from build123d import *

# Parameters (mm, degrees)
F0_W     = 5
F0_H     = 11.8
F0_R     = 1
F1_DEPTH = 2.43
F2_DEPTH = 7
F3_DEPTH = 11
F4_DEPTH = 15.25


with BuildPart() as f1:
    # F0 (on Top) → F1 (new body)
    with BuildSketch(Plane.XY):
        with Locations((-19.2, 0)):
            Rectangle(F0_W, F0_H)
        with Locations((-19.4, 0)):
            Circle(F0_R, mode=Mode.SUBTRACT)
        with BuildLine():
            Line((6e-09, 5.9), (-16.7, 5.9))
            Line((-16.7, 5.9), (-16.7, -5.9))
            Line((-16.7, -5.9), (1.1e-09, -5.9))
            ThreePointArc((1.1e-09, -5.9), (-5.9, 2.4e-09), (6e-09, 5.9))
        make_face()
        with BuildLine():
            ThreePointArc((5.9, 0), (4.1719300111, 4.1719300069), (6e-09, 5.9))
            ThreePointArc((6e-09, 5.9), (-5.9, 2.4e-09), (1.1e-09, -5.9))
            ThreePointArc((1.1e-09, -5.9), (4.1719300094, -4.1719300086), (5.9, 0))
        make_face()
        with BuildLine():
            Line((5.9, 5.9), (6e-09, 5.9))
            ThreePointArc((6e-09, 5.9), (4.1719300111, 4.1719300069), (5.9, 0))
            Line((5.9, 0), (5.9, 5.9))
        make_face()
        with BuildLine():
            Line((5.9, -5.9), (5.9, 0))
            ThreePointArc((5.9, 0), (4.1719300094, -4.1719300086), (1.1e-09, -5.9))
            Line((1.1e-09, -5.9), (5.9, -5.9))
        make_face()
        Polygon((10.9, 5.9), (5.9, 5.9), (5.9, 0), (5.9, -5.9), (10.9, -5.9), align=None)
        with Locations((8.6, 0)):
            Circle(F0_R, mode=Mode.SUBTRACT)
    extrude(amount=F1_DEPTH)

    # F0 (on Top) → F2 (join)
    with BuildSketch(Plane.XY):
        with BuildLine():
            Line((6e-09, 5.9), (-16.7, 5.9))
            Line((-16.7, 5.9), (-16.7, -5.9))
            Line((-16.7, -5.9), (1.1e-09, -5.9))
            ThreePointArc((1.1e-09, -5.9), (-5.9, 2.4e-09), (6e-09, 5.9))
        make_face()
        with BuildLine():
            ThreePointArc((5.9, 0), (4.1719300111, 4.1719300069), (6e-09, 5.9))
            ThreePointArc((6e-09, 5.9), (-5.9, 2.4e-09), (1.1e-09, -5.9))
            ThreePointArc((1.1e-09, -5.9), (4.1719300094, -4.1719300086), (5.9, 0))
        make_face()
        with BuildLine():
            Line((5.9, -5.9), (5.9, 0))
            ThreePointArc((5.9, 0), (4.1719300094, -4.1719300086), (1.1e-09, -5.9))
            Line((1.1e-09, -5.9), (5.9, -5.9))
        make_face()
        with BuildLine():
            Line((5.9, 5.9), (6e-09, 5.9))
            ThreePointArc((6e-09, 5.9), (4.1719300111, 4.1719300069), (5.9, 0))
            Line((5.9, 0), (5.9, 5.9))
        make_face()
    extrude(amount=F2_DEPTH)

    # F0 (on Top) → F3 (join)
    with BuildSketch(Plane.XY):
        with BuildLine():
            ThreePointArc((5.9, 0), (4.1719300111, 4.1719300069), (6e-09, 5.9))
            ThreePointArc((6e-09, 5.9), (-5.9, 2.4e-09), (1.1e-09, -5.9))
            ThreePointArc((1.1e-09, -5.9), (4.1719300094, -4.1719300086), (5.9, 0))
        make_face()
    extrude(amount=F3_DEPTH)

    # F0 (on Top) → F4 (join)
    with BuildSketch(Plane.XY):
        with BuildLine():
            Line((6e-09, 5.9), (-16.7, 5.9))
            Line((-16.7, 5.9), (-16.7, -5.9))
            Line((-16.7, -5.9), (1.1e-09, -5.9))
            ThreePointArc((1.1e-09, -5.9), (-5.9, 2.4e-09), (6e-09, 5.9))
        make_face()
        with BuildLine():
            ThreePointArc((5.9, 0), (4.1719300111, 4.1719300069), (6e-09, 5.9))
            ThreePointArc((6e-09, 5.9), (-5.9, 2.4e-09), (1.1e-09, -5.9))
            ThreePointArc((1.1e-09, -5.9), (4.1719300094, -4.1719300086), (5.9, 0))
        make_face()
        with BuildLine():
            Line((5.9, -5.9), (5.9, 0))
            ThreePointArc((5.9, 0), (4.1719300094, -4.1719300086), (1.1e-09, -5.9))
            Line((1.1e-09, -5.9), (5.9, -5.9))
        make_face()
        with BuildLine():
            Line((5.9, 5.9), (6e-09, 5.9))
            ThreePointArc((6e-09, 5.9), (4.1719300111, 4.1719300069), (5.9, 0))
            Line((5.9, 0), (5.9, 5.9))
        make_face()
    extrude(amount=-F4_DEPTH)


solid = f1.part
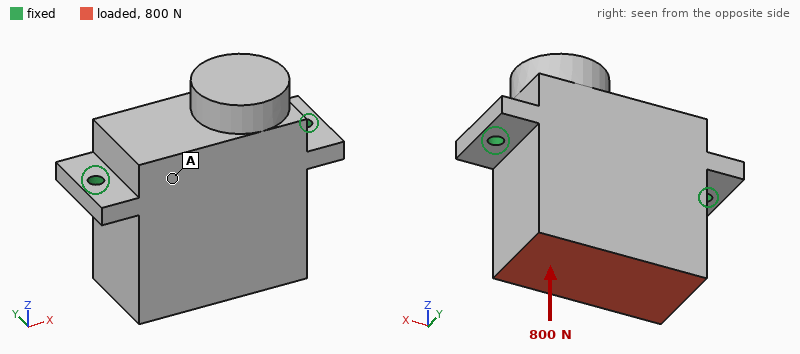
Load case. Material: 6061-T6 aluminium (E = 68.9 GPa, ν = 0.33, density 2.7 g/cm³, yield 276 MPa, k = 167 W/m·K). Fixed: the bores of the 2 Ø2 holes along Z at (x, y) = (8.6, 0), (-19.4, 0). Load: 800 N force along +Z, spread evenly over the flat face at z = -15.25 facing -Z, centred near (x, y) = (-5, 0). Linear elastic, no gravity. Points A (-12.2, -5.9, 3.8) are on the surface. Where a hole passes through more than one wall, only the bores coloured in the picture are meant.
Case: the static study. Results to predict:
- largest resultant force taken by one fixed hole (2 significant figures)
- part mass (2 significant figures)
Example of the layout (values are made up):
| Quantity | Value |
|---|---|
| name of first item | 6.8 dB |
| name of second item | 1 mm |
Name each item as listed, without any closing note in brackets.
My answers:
| Quantity | Value |
|---|---|
| largest resultant force taken by one fixed hole | 400 N |
| part mass | 18 g |
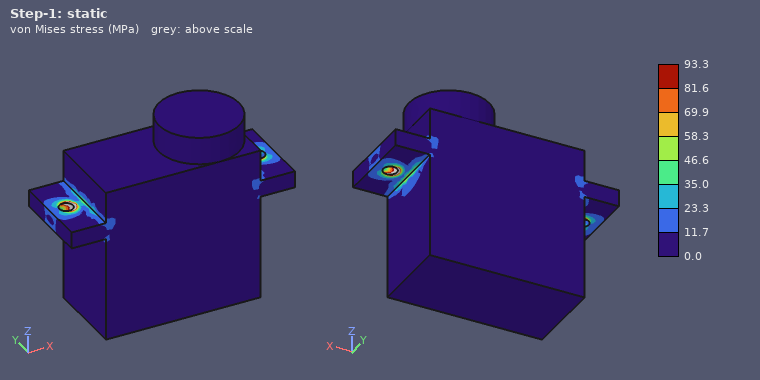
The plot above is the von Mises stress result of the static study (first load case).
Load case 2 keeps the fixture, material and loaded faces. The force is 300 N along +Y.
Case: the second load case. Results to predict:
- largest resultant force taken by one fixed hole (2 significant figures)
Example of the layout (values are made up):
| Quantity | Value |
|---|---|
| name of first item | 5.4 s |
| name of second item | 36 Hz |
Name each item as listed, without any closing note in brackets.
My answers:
| Quantity | Value |
|---|---|
| largest resultant force taken by one fixed hole | 150 N |
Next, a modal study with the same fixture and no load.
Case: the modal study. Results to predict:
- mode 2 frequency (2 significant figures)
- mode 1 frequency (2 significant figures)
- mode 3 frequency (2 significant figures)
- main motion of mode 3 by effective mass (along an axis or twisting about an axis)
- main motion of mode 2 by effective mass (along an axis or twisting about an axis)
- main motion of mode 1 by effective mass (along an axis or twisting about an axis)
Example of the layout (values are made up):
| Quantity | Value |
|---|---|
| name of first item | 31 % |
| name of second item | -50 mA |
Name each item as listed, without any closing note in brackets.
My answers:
| Quantity | Value |
|---|---|
| mode 2 frequency | 14 kHz |
| mode 1 frequency | 3900 Hz |
| mode 3 frequency | 16 kHz |
| main motion of mode 3 by effective mass | along X |
| main motion of mode 2 by effective mass | along Z |
| main motion of mode 1 by effective mass | along Y |
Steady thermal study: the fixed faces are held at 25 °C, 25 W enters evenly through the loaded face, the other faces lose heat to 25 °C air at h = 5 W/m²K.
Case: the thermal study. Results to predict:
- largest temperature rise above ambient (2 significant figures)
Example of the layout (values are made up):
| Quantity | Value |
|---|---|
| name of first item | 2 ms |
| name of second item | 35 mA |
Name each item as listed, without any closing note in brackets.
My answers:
| Quantity | Value |
|---|---|
| largest temperature rise above ambient | 23 K |
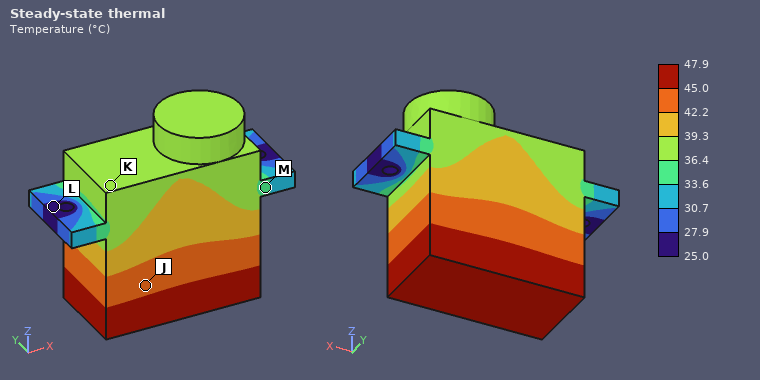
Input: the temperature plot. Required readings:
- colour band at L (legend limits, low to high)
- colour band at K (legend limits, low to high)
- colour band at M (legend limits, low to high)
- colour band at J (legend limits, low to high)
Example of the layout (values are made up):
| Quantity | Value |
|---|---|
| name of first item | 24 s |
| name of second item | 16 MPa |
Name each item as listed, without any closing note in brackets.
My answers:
| Quantity | Value |
|---|---|
| colour band at L | 25.0 to 27.9 °C |
| colour band at K | 36.4 to 39.3 °C |
| colour band at M | 33.6 to 36.4 °C |
| colour band at J | 42.2 to 45.0 °C |
